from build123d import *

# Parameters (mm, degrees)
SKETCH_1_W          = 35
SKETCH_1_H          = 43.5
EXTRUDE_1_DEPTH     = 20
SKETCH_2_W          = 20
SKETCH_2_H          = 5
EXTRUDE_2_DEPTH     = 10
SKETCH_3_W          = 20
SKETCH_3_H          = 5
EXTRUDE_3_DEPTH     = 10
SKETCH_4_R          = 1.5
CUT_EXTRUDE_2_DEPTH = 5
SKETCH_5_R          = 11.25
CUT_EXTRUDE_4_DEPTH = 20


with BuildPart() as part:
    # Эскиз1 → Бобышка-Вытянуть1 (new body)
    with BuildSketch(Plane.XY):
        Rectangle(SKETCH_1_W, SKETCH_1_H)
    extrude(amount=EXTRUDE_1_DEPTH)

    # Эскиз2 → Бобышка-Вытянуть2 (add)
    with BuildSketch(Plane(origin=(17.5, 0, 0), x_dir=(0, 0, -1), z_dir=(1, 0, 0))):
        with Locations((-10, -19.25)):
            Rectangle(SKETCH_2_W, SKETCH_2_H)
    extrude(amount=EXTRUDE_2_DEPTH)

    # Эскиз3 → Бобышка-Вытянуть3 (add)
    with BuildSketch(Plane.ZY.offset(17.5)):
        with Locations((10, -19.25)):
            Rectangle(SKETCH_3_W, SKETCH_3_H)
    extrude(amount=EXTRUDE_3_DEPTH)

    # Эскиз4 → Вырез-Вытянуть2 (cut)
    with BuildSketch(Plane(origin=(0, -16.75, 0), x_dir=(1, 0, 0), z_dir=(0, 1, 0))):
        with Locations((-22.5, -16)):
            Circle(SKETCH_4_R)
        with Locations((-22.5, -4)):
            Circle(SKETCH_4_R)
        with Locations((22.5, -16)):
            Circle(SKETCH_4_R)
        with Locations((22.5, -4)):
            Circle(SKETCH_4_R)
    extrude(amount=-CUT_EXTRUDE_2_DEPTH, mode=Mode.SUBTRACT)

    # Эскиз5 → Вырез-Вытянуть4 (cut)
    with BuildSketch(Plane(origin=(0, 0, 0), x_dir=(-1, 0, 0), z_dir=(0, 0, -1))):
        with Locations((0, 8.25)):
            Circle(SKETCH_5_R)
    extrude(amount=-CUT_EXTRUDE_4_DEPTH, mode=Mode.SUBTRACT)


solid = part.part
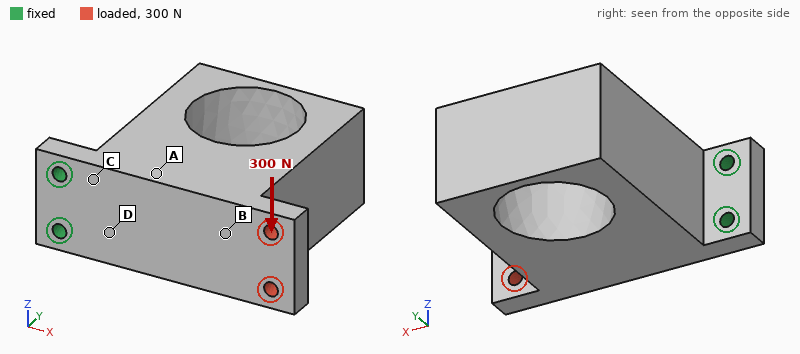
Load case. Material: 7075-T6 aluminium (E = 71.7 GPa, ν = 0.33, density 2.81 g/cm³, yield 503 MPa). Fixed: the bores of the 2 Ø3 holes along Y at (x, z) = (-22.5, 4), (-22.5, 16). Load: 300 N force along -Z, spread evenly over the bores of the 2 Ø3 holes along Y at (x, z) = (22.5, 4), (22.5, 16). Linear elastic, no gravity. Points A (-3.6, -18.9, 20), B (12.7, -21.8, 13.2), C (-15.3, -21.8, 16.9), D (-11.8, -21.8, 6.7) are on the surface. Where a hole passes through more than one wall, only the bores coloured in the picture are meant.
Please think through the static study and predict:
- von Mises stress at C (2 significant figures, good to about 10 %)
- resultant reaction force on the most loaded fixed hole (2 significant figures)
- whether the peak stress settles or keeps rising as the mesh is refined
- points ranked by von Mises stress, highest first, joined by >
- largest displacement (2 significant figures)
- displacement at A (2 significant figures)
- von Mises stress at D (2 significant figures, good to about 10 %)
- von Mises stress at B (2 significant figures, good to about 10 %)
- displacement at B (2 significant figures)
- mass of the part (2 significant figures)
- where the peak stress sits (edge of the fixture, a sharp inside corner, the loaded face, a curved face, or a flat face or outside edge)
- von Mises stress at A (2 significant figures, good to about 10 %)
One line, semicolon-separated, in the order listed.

23 MPa; 1.0 kN; keeps rising; C > D > A > B; 39 µm; 13 µm; 15 MPa; 4.0 MPa; 24 µm; 68 g; edge of the fixture; 9.3 MPa
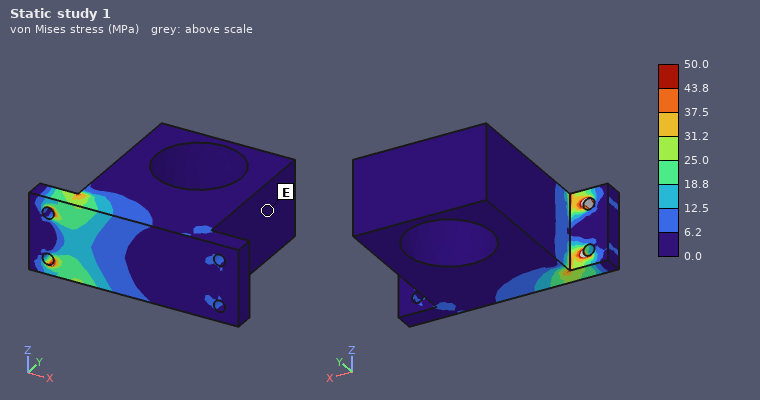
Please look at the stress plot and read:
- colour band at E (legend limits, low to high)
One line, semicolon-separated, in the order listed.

0.0 to 6.2 MPa
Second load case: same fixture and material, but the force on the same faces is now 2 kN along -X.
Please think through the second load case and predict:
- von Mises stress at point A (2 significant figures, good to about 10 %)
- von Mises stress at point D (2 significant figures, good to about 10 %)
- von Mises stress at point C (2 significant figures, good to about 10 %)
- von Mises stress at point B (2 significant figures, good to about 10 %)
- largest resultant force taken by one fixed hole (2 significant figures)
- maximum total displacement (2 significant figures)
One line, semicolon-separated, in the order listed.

13 MPa; 21 MPa; 25 MPa; 21 MPa; 1.0 kN; 27 µm
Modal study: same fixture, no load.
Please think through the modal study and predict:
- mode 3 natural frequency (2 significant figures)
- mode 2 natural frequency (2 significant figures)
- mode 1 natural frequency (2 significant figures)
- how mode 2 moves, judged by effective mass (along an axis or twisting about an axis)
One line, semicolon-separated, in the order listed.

4400 Hz; 2400 Hz; 900 Hz; along Z
